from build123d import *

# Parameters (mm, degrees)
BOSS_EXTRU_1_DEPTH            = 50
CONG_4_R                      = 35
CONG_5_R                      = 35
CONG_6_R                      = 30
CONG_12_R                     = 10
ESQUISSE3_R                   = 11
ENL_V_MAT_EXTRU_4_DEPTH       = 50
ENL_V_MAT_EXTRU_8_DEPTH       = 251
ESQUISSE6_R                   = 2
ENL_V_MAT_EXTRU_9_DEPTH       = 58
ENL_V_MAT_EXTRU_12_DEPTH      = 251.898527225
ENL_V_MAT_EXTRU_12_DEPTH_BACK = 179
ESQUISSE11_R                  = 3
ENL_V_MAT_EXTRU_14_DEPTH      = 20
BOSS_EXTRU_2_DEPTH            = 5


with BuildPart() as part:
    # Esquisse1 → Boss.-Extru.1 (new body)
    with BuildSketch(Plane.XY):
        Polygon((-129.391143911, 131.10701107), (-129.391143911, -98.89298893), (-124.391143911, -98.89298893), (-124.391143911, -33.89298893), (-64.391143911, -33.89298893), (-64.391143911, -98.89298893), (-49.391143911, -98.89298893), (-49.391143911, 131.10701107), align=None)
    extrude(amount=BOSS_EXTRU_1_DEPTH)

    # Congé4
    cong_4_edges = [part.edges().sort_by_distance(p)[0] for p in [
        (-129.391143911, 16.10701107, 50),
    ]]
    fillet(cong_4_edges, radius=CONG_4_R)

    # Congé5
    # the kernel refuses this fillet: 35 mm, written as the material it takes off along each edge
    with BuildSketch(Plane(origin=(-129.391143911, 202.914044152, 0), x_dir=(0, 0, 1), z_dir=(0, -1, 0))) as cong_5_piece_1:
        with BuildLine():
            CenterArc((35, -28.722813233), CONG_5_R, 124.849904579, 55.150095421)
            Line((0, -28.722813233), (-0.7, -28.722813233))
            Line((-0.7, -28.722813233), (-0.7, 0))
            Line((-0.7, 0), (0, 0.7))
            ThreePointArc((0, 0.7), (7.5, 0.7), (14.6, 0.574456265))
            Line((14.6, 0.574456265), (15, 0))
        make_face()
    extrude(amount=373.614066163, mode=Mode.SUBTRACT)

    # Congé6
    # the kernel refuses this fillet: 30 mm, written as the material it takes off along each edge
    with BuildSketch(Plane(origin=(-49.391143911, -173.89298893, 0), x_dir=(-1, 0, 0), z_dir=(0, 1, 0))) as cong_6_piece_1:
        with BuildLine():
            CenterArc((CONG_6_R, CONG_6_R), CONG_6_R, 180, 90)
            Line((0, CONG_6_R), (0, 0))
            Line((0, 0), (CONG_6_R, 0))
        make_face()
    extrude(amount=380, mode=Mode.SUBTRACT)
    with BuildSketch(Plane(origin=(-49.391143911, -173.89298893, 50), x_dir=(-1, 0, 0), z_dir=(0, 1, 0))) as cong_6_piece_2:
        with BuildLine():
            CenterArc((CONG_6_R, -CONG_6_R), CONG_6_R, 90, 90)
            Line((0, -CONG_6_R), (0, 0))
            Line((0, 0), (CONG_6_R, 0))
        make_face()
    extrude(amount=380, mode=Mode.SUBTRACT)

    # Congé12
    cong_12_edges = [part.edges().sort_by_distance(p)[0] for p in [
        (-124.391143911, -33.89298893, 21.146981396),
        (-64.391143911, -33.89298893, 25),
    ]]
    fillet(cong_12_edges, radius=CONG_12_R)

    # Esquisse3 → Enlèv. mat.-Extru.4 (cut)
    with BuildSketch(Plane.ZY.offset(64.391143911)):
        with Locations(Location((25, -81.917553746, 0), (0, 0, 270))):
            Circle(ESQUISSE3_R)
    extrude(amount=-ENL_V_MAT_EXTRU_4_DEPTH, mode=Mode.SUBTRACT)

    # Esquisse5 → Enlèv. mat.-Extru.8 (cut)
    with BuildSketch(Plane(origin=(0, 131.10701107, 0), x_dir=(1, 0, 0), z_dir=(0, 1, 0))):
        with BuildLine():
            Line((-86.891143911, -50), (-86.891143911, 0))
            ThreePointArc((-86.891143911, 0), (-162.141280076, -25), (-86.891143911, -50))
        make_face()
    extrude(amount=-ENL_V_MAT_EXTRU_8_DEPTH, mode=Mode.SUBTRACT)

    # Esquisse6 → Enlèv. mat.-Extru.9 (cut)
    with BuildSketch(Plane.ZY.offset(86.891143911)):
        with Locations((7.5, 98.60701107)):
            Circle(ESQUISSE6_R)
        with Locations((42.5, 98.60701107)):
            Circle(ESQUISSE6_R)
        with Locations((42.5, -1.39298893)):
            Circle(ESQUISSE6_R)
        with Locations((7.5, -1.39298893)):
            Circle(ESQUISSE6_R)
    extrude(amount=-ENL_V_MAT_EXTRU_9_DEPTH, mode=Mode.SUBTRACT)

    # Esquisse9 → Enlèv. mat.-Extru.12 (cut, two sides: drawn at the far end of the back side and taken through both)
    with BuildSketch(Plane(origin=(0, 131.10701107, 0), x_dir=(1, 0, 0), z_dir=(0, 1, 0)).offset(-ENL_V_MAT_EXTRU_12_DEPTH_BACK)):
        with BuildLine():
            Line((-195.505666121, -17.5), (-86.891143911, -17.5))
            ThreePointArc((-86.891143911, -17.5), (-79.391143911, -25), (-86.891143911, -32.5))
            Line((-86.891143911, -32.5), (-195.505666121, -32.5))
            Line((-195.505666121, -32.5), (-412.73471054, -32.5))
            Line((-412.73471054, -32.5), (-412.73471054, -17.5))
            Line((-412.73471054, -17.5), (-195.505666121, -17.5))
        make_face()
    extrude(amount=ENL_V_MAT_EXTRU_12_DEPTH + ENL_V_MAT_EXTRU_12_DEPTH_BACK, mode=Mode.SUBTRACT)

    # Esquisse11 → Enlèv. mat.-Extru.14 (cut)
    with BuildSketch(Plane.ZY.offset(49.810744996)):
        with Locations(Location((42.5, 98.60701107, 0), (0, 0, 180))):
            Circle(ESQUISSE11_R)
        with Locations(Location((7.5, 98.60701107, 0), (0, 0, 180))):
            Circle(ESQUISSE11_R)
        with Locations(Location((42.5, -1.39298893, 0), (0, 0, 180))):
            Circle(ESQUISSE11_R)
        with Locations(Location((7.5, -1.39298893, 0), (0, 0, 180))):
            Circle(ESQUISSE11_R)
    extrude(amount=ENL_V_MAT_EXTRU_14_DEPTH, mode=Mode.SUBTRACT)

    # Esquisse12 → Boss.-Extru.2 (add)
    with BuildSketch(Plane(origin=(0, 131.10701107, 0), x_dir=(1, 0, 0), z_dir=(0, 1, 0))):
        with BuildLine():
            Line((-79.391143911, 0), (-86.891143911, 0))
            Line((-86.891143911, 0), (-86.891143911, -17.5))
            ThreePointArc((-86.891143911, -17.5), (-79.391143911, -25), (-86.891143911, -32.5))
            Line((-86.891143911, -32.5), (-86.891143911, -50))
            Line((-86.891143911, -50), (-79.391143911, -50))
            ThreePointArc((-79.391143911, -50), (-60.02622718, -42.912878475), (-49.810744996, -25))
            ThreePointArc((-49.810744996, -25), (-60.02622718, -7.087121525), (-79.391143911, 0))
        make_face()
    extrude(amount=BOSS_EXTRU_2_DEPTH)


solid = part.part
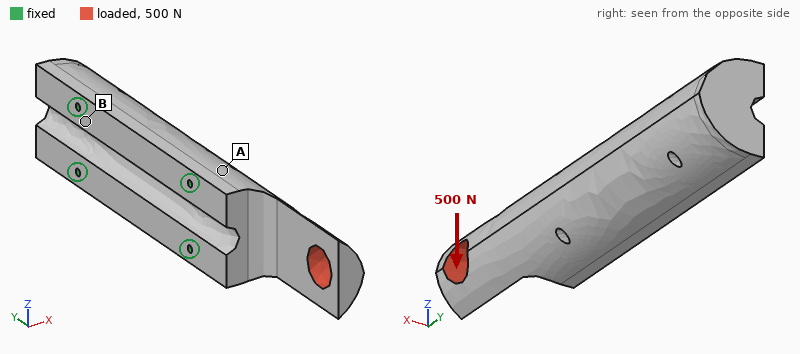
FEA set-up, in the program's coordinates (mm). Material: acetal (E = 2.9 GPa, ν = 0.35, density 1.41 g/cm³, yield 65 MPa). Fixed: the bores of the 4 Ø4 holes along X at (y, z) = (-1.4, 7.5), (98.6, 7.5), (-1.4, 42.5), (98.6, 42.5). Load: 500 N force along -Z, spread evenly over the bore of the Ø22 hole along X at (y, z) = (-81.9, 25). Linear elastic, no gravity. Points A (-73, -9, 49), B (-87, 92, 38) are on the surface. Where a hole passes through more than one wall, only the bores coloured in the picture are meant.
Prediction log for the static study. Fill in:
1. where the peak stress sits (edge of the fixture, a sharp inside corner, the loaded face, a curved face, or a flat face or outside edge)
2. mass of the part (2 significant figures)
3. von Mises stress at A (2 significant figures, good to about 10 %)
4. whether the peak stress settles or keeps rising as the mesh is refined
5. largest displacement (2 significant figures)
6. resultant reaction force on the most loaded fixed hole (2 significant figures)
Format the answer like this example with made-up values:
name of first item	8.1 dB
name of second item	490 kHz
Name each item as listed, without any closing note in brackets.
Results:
where the peak stress sits	edge of the fixture
mass of the part	360 g
von Mises stress at A	3.6 MPa
whether the peak stress settles or keeps rising as the mesh is refined	keeps rising
largest displacement	0.79 mm
resultant reaction force on the most loaded fixed hole	1.0 kN
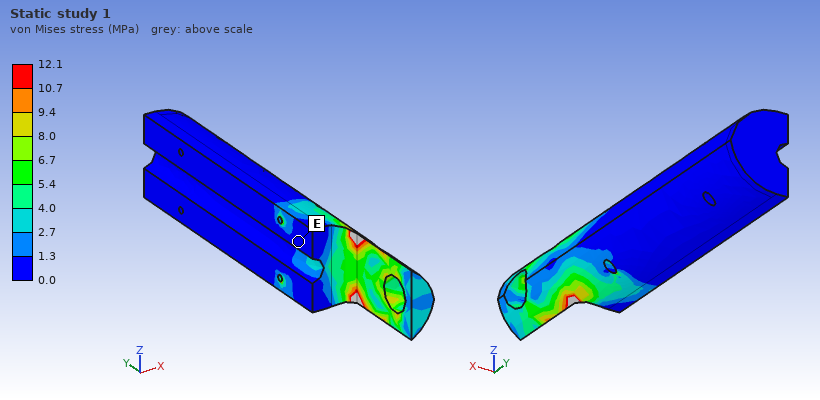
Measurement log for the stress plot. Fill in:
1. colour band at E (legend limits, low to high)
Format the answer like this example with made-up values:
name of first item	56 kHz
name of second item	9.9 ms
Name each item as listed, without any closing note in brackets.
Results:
colour band at E	0.0 to 1.3 MPa
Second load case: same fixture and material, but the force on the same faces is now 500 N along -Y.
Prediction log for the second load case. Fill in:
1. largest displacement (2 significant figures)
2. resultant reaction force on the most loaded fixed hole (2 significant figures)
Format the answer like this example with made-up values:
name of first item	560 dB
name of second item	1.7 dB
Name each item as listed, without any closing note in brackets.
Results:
largest displacement	0.27 mm
resultant reaction force on the most loaded fixed hole	160 N
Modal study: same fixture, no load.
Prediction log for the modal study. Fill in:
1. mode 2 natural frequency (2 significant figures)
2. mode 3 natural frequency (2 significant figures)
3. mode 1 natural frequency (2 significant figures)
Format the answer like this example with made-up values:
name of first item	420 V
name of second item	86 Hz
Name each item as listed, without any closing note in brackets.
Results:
mode 2 natural frequency	1200 Hz
mode 3 natural frequency	1800 Hz
mode 1 natural frequency	660 Hz
